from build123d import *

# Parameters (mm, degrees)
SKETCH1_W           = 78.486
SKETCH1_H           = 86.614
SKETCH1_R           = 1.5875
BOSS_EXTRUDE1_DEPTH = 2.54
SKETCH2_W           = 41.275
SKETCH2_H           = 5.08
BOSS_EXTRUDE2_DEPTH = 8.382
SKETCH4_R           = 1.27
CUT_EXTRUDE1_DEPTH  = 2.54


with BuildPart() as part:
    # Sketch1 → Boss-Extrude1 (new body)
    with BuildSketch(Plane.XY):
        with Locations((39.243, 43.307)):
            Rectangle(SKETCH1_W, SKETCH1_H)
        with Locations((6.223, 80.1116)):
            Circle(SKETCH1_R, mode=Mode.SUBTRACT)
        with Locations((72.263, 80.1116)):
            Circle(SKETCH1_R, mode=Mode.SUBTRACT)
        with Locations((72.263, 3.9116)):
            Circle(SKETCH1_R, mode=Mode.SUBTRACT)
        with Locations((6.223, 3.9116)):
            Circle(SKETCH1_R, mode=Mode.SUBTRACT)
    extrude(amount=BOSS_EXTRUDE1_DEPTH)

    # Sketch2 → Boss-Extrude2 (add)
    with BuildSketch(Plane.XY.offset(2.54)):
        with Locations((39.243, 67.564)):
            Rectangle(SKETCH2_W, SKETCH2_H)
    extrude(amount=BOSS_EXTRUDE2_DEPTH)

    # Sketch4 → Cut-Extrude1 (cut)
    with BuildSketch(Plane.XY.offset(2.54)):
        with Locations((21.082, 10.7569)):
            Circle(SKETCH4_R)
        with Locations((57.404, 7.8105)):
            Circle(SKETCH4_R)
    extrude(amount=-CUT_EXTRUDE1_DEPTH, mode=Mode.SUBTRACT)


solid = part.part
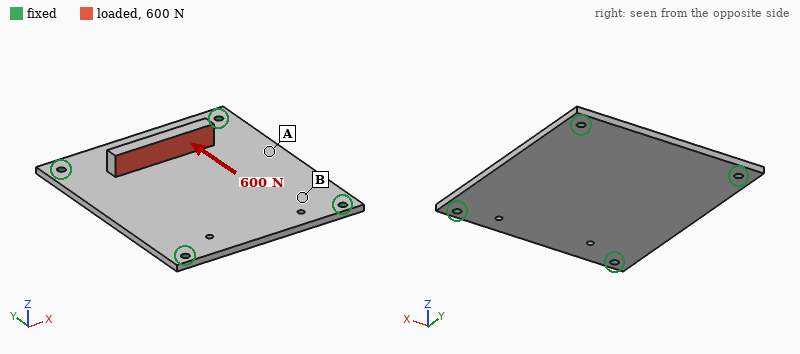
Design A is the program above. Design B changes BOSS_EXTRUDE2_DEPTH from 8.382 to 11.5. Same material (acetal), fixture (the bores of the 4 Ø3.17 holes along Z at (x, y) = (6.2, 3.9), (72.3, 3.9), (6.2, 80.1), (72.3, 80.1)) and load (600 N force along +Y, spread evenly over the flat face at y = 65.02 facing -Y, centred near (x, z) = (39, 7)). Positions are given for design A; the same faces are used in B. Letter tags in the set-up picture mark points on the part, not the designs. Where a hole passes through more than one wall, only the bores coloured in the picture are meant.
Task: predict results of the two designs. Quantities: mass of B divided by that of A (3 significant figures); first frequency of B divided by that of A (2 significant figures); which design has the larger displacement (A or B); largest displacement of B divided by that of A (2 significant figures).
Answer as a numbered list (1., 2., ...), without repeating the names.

1. 1.03
2. 0.99
3. B
4. 1.4
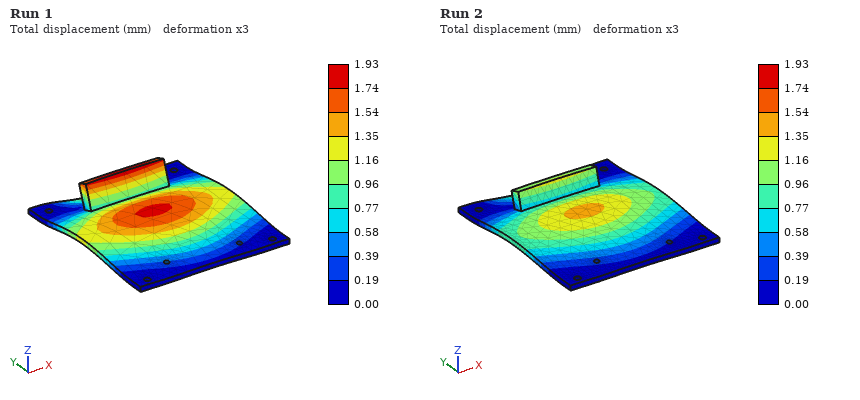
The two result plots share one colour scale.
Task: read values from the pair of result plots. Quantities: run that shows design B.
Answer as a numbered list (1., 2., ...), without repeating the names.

1. Run 1
